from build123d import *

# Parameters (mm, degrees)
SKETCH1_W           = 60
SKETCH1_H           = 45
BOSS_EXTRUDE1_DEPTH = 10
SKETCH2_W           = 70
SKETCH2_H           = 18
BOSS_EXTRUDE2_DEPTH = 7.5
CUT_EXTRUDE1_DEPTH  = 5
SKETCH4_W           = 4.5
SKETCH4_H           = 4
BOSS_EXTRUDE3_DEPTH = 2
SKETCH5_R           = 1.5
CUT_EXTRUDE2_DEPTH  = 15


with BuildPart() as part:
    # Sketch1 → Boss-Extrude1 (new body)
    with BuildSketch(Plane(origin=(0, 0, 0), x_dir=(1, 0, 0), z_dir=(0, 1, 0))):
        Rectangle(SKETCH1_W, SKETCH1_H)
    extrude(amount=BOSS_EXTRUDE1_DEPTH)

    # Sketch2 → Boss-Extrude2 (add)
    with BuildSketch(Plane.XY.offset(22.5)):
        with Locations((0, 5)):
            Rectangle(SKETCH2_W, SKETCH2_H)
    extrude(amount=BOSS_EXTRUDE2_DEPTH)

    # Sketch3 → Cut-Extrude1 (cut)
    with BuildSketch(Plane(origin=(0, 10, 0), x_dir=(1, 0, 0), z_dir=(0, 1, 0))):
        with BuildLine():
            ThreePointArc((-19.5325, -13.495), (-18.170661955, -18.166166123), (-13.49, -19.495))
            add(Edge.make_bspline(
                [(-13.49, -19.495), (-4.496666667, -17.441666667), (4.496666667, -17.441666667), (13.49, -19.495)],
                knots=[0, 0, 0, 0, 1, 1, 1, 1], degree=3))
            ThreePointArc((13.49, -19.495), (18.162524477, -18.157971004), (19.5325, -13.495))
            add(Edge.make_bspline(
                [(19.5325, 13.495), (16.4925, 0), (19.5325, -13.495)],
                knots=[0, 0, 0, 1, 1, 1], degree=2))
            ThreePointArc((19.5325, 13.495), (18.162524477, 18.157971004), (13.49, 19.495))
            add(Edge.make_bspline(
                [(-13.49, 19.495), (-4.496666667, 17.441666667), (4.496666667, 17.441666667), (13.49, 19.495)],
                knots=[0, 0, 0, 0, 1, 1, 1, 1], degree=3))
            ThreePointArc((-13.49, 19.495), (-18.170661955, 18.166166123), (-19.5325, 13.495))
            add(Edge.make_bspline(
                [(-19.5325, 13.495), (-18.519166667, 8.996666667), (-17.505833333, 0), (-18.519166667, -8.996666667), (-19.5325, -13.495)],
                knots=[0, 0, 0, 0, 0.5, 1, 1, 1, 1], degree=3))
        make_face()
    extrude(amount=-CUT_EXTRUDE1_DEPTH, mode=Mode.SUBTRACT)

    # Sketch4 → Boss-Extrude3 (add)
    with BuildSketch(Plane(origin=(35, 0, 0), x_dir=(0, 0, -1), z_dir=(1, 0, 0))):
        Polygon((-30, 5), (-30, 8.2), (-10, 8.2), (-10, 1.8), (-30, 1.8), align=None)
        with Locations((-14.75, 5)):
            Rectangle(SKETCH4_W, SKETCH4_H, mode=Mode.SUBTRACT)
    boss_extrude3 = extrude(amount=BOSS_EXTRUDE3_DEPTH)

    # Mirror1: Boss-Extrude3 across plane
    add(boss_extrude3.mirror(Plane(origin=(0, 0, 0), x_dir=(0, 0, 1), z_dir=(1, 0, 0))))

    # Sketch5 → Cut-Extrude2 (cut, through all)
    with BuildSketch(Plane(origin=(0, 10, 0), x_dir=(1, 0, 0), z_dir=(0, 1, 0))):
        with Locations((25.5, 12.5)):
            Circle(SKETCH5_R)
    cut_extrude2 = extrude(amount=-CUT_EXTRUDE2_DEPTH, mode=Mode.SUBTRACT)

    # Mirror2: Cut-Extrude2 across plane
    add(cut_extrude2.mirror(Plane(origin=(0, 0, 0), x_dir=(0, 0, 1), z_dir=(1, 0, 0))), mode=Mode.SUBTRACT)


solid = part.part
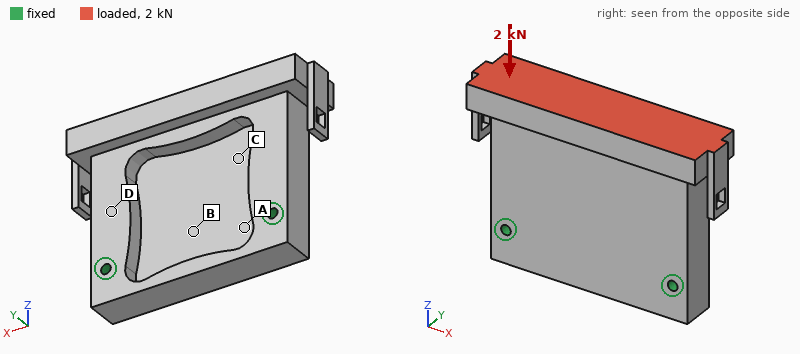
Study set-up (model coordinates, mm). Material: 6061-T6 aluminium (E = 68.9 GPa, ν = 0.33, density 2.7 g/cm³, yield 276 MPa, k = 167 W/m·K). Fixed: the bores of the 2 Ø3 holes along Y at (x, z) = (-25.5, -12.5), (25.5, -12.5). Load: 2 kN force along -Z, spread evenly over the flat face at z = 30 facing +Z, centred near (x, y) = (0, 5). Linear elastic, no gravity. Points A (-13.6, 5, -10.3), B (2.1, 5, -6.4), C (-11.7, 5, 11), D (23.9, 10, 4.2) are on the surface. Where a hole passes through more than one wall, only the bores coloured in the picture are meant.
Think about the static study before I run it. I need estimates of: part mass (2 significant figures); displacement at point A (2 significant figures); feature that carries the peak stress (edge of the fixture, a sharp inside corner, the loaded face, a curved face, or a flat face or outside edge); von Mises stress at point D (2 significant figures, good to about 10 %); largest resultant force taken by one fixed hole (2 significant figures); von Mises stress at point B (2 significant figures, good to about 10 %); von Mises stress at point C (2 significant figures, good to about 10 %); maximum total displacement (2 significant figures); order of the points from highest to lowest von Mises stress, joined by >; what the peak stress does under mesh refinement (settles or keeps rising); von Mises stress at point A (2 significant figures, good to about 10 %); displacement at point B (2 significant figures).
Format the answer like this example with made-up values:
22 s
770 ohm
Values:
80 g
1.8 µm
edge of the fixture
9.2 MPa
1.0 kN
2.0 MPa
6.0 MPa
10.0 µm
D > C > A > B
keeps rising
3.1 MPa
2.5 µm
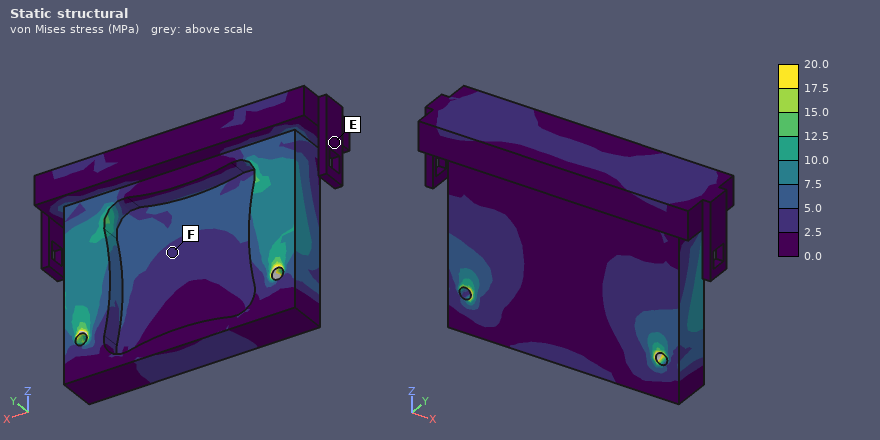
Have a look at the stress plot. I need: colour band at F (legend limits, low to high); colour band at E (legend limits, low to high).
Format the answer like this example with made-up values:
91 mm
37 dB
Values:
2.5 to 5.0 MPa
0.0 to 2.5 MPa
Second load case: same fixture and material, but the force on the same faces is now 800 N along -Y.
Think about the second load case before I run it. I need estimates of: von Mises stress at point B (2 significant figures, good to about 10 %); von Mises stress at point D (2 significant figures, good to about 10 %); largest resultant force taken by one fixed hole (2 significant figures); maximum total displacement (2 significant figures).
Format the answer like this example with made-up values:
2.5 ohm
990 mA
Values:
18 MPa
43 MPa
400 N
0.15 mm
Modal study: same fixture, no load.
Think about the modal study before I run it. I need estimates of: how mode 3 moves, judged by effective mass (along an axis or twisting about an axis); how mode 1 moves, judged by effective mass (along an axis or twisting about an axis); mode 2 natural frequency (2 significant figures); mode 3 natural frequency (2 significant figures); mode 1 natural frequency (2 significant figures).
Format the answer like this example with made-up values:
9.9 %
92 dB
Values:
along X
along Y
4300 Hz
9000 Hz
2300 Hz
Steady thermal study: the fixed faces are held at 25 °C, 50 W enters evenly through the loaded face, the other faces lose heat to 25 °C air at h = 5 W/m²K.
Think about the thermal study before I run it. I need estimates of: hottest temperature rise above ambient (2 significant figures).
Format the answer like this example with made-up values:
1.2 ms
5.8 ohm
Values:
32 K
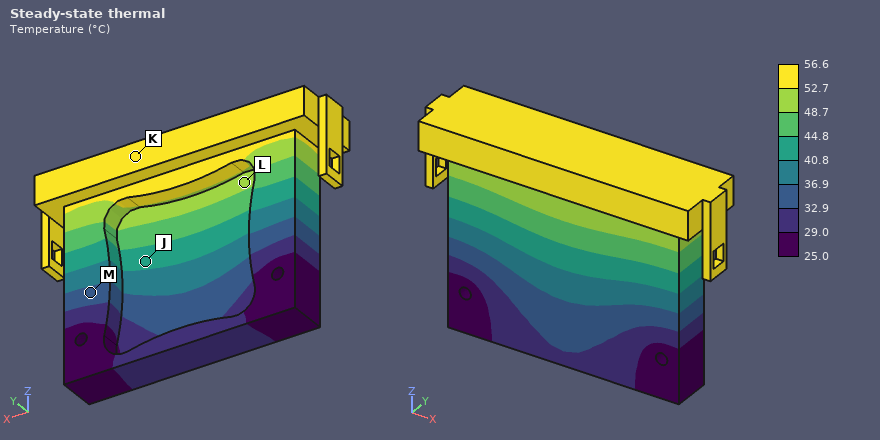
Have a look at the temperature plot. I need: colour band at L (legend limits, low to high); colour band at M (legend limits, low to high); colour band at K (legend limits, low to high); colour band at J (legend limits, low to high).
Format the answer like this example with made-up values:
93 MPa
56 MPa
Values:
48.7 to 52.7 °C
32.9 to 36.9 °C
52.7 to 56.6 °C
40.8 to 44.8 °C
